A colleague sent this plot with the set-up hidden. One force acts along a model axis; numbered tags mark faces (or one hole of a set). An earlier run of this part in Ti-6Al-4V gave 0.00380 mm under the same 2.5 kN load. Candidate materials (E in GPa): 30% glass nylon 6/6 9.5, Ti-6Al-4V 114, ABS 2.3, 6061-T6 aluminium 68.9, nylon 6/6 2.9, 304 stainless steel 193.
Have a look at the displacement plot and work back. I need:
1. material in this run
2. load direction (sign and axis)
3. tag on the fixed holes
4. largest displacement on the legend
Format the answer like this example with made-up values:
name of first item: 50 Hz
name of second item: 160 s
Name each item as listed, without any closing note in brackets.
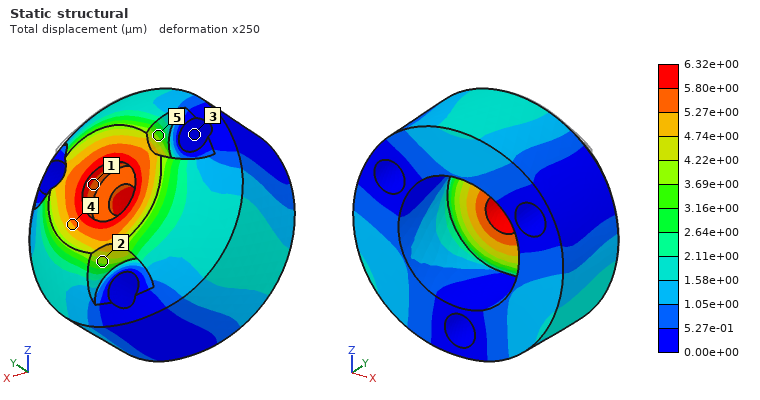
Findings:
material in this run: 6061-T6 aluminium
load direction: -Y
tag on the fixed holes: 3
largest displacement on the legend: 6.32e+00 µm
